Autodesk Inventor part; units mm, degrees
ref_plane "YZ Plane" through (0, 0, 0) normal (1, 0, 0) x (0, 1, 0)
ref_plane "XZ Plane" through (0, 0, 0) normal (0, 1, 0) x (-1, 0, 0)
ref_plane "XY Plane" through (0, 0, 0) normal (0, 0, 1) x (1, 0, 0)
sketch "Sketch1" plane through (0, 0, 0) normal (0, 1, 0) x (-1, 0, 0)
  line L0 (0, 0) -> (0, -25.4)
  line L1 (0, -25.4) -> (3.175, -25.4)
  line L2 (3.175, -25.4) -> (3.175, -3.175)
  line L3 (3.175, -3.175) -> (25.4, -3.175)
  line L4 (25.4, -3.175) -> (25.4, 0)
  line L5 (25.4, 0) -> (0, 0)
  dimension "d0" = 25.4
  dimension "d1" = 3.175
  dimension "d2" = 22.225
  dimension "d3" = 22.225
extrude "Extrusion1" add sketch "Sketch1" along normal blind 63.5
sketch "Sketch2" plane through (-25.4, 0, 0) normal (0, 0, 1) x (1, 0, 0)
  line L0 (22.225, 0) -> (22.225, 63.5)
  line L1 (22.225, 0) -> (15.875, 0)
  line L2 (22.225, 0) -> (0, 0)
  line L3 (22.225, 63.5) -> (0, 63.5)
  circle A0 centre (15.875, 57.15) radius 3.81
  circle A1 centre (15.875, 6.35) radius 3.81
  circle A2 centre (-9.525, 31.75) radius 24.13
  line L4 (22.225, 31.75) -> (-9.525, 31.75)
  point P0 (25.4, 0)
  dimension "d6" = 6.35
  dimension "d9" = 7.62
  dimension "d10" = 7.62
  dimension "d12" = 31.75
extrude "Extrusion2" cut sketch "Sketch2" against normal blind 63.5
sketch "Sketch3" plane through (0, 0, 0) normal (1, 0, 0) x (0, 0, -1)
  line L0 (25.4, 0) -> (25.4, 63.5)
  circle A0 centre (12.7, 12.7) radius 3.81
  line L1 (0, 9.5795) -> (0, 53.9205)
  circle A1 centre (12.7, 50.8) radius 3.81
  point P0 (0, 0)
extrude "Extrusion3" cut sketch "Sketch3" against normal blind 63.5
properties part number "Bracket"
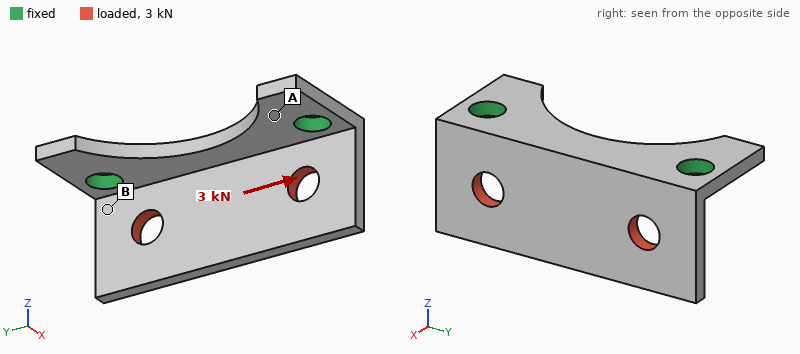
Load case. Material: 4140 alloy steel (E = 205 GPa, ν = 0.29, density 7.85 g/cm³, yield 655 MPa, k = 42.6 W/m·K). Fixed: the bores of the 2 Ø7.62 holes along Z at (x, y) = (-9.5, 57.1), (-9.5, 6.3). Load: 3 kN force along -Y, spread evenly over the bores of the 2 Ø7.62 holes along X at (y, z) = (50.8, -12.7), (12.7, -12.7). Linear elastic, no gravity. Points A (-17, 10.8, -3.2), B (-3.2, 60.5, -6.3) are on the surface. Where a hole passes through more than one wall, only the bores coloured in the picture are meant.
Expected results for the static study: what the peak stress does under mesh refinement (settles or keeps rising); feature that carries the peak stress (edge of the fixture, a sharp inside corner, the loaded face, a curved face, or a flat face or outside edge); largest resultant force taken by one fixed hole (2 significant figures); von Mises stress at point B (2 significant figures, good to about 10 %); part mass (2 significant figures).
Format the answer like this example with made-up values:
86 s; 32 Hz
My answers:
keeps rising; edge of the fixture; 1.7 kN; 35 MPa; 59 g
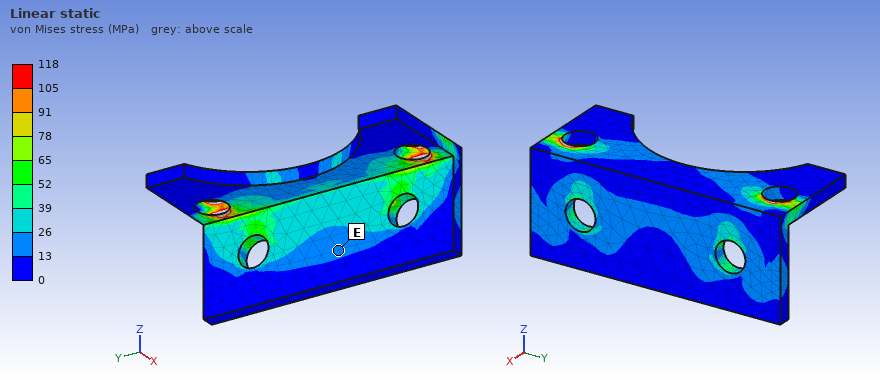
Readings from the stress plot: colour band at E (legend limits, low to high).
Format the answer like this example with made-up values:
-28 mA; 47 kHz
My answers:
13 to 26 MPa
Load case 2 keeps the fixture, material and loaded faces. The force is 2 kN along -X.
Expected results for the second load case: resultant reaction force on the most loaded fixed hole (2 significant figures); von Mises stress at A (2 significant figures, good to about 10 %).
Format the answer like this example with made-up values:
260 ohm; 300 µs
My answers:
1.0 kN; 48 MPa
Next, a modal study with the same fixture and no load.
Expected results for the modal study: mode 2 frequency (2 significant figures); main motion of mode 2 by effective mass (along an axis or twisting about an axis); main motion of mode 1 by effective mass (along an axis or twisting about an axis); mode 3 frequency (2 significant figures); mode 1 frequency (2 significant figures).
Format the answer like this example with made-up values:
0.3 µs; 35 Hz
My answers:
5000 Hz; twisting about Z; along X; 8500 Hz; 3100 Hz
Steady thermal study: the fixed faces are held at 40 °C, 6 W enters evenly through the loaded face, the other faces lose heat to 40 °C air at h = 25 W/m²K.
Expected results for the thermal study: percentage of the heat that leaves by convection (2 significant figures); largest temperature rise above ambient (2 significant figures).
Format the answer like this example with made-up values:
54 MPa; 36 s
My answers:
18 %; 16 K
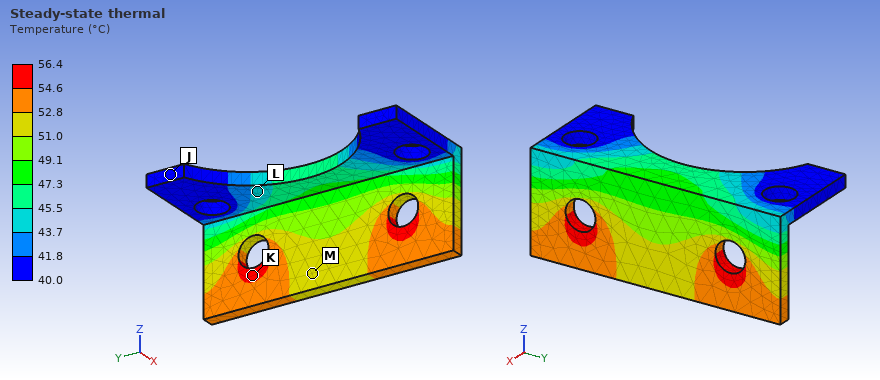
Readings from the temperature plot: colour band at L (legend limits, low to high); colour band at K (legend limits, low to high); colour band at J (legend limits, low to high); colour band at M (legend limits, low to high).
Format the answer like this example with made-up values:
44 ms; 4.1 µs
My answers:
43.7 to 45.5 °C; 54.6 to 56.4 °C; 40.0 to 41.8 °C; 51.0 to 52.8 °C
